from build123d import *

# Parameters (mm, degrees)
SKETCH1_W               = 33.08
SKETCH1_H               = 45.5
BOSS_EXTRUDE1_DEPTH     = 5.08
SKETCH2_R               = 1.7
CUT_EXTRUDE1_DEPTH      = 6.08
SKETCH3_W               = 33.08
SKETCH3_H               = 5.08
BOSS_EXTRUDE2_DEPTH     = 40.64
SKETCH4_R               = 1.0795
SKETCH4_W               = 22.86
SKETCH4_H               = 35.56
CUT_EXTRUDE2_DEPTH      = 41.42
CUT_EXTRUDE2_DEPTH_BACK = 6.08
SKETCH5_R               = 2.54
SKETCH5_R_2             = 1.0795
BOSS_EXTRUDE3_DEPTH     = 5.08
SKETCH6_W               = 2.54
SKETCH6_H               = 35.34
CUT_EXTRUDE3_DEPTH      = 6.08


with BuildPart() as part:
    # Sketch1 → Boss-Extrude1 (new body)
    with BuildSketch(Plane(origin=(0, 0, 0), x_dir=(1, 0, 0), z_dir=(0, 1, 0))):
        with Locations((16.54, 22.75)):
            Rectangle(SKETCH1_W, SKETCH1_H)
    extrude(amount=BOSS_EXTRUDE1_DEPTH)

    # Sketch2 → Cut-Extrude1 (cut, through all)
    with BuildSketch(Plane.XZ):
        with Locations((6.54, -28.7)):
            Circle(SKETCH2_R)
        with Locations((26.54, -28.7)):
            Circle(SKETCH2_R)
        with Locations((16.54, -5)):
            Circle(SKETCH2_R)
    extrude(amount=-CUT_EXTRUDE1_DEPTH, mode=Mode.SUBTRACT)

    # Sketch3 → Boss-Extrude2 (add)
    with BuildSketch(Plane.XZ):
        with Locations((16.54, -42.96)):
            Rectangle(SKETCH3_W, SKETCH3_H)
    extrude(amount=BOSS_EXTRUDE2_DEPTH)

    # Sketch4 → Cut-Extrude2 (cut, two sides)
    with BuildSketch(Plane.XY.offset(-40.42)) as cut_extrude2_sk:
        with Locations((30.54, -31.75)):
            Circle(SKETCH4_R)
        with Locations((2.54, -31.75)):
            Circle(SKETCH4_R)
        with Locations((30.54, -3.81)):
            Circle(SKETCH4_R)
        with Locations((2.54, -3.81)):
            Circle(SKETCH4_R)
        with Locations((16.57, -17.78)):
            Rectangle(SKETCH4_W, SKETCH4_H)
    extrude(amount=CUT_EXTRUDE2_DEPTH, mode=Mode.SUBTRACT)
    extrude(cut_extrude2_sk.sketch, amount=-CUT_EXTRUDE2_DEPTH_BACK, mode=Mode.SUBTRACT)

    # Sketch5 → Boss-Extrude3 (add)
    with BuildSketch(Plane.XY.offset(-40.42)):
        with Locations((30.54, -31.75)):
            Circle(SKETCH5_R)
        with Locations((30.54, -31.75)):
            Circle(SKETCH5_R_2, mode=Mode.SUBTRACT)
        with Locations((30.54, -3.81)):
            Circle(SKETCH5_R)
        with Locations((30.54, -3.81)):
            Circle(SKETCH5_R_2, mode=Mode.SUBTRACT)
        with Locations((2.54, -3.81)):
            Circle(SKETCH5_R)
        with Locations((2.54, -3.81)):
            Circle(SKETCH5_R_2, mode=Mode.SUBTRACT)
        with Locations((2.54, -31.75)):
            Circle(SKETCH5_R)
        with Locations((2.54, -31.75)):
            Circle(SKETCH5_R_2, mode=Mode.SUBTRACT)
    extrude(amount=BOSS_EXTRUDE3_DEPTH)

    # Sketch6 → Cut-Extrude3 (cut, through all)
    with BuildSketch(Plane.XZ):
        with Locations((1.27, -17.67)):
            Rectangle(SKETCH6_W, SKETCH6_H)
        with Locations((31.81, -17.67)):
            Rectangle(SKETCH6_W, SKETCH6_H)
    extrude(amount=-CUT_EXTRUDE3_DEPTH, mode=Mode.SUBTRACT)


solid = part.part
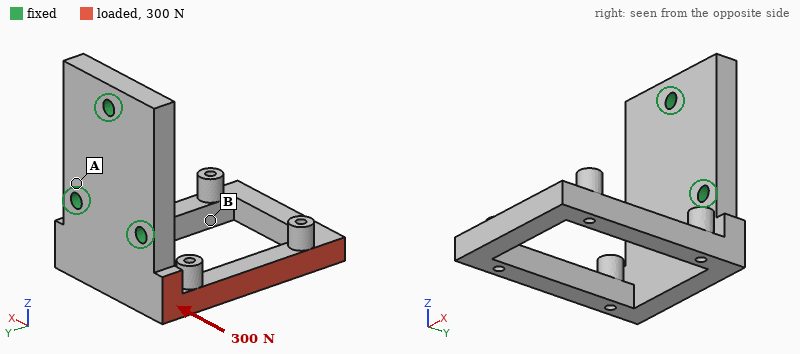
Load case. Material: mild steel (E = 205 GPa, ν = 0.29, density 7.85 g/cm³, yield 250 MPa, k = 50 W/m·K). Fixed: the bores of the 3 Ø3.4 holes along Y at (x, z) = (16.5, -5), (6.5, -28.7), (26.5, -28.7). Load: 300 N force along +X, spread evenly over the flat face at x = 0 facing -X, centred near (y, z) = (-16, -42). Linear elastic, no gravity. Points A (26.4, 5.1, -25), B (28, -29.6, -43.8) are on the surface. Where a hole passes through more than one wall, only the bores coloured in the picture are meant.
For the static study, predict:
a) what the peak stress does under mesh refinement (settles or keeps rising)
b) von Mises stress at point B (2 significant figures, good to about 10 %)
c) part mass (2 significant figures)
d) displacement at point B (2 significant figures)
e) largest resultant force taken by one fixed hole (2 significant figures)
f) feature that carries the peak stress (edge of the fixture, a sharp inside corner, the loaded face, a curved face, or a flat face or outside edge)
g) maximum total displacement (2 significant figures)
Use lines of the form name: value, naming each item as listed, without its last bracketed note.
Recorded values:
what the peak stress does under mesh refinement: keeps rising
von Mises stress at point B: 30 MPa
part mass: 75 g
displacement at point B: 50 µm
largest resultant force taken by one fixed hole: 330 N
feature that carries the peak stress: a sharp inside corner
maximum total displacement: 64 µm
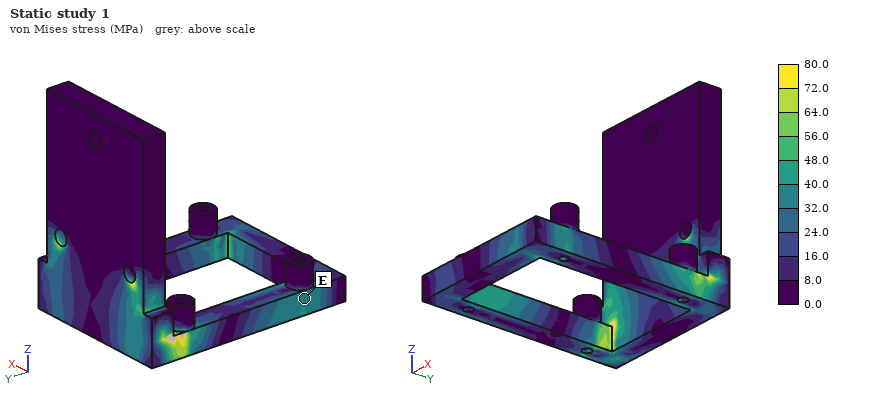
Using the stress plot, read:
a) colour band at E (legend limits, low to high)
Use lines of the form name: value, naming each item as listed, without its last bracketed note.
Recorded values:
colour band at E: 32.0 to 40.0 MPa
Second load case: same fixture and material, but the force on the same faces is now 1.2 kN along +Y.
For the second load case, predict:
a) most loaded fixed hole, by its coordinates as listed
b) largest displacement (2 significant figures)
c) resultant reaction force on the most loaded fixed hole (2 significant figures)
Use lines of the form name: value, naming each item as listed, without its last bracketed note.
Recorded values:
most loaded fixed hole, by its coordinates as listed: (6.5, -28.7)
largest displacement: 0.15 mm
resultant reaction force on the most loaded fixed hole: 1.5 kN
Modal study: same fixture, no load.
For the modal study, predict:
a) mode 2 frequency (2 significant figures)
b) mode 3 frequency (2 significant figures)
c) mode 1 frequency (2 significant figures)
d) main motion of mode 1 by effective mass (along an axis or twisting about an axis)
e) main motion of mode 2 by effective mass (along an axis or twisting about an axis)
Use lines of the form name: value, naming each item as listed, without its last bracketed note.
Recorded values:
mode 2 frequency: 2100 Hz
mode 3 frequency: 3300 Hz
mode 1 frequency: 1300 Hz
main motion of mode 1 by effective mass: along Z
main motion of mode 2 by effective mass: along X
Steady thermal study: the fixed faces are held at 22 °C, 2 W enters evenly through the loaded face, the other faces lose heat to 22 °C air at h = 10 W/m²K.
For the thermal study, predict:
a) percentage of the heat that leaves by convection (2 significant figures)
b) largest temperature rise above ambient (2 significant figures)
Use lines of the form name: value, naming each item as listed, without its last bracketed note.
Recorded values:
percentage of the heat that leaves by convection: 16 %
largest temperature rise above ambient: 19 K
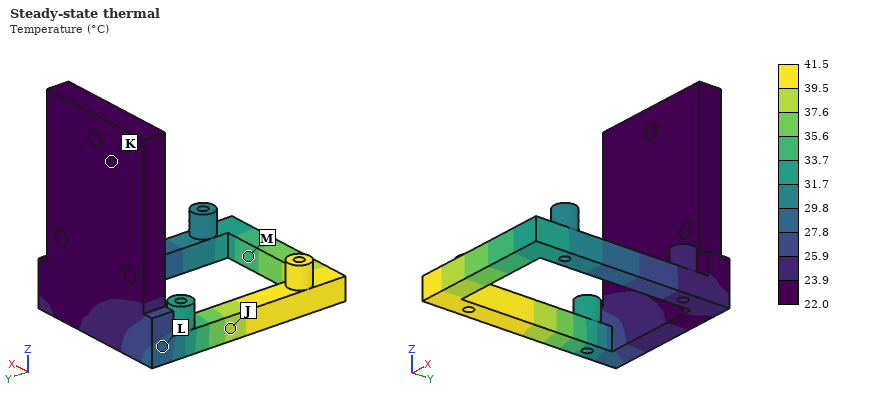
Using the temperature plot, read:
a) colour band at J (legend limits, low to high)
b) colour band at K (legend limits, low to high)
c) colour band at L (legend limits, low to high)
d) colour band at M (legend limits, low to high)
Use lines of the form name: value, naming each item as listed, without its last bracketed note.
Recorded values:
colour band at J: 37.6 to 39.5 °C
colour band at K: 22.0 to 23.9 °C
colour band at L: 27.8 to 29.8 °C
colour band at M: 33.7 to 35.6 °C
